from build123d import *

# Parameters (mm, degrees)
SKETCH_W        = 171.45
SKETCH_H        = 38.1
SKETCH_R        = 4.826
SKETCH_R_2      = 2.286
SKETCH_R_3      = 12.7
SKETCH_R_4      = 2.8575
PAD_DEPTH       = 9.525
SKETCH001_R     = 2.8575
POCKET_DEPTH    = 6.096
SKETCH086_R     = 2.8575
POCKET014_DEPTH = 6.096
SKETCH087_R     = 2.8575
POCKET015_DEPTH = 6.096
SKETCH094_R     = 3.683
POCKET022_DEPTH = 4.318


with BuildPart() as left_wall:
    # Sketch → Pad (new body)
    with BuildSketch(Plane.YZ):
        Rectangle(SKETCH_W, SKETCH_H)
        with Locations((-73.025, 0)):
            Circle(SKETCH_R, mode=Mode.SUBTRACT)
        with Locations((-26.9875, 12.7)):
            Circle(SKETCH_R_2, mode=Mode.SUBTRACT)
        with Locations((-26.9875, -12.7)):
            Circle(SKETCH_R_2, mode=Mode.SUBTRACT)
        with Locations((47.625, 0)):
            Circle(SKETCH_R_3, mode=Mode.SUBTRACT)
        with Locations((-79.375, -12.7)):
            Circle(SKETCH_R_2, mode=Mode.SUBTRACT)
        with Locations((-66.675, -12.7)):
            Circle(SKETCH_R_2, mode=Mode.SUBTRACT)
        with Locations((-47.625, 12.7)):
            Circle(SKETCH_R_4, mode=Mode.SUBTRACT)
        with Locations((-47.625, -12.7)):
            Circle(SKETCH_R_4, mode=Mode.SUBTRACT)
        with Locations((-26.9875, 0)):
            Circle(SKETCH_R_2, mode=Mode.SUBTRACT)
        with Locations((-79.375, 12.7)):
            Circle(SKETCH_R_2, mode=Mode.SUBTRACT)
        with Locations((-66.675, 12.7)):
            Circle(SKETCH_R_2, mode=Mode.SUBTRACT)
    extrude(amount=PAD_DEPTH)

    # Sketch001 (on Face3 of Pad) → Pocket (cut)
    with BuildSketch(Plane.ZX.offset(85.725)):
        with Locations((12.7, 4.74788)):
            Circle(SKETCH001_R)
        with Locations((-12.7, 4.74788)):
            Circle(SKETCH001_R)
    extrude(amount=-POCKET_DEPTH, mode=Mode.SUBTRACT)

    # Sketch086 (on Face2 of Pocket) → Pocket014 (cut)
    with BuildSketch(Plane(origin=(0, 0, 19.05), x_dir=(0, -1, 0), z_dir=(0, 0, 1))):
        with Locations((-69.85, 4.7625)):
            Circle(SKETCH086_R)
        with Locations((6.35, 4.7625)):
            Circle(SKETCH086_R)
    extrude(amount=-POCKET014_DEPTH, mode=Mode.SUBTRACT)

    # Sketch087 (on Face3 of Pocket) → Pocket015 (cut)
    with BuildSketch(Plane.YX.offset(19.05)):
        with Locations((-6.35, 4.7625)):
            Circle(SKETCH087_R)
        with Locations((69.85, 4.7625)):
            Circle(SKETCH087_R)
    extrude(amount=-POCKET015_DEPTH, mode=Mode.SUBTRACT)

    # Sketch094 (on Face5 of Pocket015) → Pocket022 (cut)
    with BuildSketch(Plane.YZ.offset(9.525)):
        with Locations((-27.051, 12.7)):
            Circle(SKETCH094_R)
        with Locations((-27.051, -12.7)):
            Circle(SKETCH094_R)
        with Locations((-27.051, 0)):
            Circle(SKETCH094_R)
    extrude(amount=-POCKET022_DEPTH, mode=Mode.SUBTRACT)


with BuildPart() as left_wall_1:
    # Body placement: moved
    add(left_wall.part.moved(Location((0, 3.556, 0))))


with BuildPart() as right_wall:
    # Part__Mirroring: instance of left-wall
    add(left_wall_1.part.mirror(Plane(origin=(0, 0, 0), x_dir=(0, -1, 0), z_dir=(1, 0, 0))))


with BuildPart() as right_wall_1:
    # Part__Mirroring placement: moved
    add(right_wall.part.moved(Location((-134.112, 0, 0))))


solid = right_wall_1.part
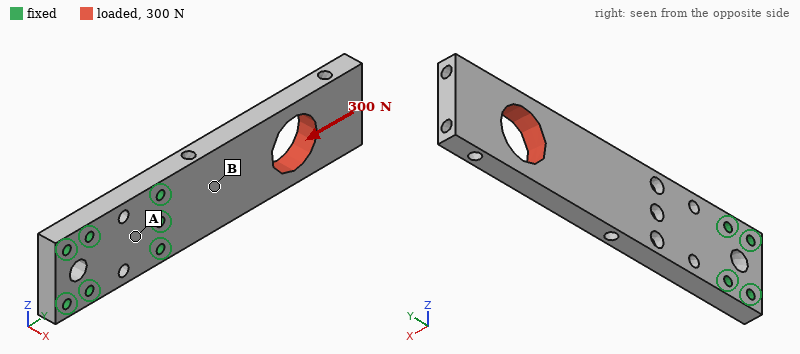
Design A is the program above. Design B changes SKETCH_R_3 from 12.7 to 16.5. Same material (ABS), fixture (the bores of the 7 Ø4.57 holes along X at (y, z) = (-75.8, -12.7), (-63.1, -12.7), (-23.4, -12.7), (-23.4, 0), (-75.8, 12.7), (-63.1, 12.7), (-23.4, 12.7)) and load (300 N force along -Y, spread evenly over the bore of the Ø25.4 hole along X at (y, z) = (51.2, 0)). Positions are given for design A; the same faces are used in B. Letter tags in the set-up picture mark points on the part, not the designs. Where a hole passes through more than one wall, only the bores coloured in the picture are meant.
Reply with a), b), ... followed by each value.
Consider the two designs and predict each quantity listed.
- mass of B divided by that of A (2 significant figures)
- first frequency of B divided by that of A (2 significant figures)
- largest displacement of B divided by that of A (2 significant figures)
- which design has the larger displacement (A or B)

a) 0.94
b) 1.0
c) 1.2
d) B
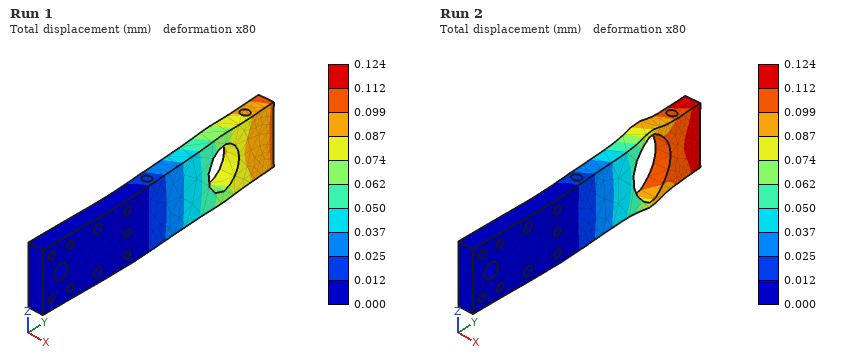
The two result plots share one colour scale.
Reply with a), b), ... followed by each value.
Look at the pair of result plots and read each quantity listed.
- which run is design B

a) Run 2
